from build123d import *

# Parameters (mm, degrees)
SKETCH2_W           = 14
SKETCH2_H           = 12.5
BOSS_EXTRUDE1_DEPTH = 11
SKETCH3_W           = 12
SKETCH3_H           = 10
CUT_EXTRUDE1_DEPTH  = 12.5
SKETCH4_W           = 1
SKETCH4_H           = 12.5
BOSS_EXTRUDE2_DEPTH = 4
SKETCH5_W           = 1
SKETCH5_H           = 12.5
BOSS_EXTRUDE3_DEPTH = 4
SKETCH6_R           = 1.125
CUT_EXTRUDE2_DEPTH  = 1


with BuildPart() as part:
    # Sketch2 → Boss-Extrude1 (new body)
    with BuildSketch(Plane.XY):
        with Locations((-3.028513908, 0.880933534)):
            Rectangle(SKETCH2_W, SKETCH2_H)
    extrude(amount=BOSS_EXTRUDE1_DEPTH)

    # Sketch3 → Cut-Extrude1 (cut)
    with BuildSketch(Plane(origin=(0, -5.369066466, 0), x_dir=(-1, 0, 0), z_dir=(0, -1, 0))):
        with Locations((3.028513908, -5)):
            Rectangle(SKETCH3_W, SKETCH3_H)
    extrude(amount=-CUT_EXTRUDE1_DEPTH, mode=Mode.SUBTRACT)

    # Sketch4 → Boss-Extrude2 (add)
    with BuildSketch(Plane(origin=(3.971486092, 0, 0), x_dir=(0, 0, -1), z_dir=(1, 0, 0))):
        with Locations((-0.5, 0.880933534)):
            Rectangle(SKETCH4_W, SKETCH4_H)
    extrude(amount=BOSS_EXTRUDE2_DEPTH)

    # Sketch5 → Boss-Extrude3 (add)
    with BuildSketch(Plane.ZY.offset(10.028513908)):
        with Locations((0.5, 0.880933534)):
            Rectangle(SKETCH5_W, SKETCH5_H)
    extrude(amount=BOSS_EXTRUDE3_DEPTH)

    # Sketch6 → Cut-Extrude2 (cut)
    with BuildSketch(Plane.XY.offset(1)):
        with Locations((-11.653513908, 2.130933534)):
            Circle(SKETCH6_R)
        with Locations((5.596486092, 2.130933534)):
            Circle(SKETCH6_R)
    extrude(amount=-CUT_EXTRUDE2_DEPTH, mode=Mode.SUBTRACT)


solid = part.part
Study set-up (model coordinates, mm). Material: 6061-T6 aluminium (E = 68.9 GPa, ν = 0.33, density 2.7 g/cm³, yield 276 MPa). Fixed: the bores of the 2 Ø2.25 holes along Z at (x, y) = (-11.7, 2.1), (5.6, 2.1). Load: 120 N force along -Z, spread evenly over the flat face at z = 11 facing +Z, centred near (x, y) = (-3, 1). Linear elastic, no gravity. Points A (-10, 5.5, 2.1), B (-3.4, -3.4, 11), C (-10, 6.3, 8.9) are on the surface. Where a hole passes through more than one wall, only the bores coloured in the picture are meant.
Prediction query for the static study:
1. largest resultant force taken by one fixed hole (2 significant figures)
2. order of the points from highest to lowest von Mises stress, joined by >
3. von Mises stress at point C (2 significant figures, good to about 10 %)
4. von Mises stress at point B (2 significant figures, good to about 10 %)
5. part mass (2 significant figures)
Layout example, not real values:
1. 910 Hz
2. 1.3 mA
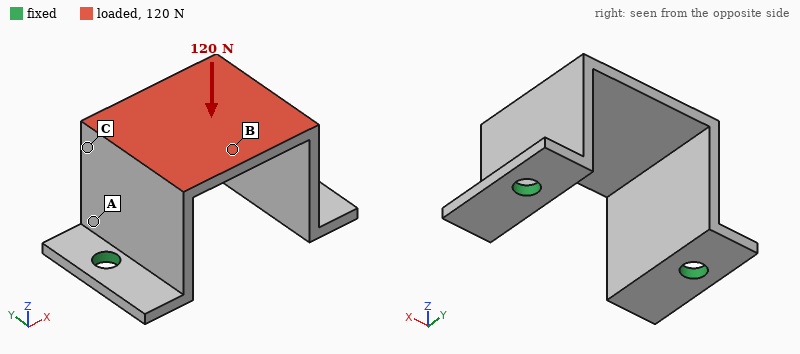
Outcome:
1. 62 N
2. B > C > A
3. 27 MPa
4. 40 MPa
5. 1.4 g
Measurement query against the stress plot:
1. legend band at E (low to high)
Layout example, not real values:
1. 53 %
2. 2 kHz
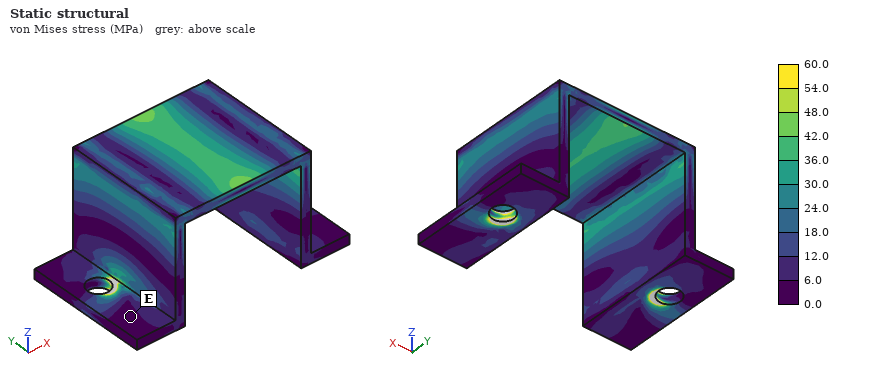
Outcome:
1. 0.0 to 6.0 MPa
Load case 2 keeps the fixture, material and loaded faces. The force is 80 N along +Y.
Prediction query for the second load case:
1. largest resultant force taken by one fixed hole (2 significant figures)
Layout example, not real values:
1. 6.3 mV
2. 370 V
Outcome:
1. 40 N
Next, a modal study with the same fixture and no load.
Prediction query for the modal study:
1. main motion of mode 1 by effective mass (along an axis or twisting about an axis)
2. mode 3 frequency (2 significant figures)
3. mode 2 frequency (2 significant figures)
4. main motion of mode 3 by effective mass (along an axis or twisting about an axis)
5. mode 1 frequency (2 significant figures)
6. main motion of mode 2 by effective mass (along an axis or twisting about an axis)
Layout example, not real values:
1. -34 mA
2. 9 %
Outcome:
1. along X
2. 9200 Hz
3. 6700 Hz
4. twisting about Z
5. 5900 Hz
6. along Y
